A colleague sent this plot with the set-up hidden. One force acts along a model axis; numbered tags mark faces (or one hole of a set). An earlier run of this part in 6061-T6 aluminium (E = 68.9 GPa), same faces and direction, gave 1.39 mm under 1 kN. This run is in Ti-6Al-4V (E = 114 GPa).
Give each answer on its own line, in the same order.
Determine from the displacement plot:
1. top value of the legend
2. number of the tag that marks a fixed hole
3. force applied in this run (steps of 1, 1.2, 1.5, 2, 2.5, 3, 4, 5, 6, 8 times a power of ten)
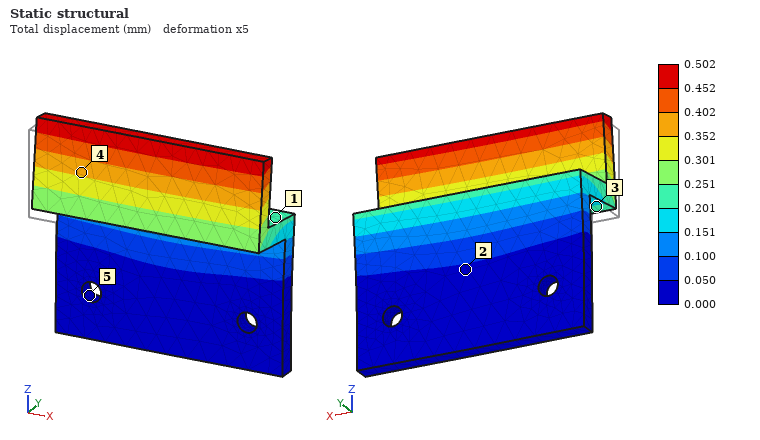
0.502 mm
5
600 N
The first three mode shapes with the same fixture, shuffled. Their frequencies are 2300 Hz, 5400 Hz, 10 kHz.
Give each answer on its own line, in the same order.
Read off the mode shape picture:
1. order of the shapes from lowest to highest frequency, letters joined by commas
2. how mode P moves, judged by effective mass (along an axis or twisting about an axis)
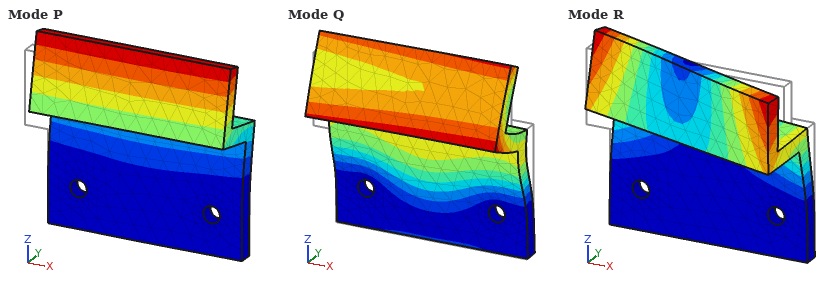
P, R, Q
along Y
